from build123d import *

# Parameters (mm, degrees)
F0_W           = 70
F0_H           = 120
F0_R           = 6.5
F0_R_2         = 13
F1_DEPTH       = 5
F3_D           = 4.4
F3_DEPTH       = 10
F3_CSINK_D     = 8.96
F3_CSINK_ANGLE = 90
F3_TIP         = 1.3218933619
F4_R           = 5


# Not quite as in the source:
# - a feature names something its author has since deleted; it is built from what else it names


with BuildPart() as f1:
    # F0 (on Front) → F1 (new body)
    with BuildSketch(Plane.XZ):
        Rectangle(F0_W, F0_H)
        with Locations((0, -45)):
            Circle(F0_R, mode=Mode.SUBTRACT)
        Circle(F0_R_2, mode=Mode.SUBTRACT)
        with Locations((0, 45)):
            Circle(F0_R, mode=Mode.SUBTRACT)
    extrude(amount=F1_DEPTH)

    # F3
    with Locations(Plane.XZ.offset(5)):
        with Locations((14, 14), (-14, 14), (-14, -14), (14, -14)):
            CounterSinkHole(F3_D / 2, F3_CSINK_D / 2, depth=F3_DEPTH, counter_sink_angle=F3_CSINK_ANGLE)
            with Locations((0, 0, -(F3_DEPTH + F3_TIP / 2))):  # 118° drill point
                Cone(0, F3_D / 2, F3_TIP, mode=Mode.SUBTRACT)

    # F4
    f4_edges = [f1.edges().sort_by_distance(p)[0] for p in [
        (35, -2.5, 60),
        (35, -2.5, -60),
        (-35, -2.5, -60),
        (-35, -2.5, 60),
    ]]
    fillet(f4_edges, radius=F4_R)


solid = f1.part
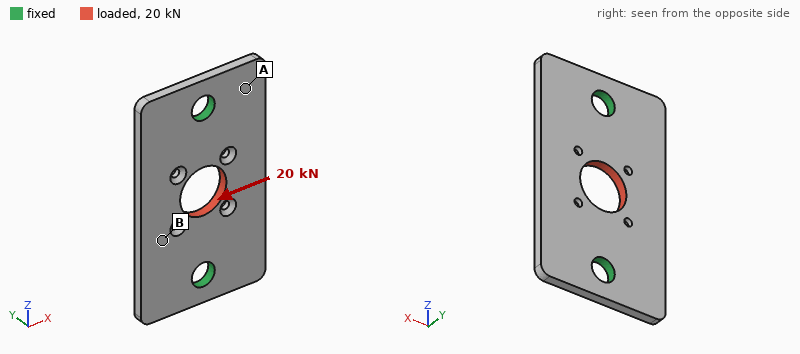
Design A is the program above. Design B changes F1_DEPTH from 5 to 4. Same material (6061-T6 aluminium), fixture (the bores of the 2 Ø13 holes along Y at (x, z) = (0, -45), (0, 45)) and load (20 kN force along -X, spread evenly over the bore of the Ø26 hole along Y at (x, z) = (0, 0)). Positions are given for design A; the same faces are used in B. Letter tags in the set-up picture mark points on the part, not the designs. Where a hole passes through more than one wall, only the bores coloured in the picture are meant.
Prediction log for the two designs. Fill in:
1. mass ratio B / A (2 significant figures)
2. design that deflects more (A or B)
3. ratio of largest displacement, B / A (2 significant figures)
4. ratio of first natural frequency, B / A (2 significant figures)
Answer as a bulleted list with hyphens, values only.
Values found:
- 0.80
- B
- 1.2
- 0.82
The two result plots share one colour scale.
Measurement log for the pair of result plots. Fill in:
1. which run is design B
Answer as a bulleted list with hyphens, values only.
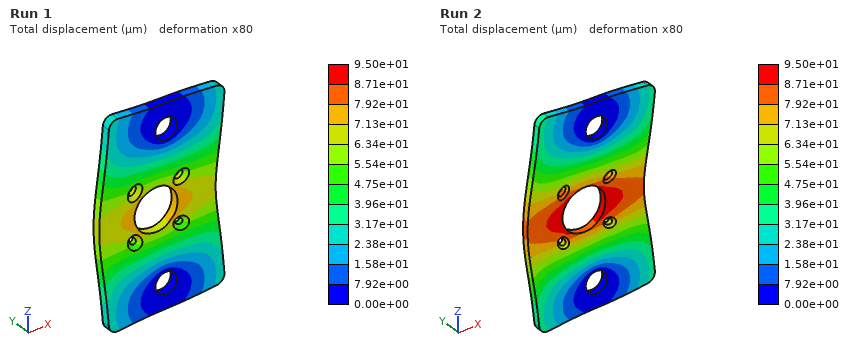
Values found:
- Run 2
